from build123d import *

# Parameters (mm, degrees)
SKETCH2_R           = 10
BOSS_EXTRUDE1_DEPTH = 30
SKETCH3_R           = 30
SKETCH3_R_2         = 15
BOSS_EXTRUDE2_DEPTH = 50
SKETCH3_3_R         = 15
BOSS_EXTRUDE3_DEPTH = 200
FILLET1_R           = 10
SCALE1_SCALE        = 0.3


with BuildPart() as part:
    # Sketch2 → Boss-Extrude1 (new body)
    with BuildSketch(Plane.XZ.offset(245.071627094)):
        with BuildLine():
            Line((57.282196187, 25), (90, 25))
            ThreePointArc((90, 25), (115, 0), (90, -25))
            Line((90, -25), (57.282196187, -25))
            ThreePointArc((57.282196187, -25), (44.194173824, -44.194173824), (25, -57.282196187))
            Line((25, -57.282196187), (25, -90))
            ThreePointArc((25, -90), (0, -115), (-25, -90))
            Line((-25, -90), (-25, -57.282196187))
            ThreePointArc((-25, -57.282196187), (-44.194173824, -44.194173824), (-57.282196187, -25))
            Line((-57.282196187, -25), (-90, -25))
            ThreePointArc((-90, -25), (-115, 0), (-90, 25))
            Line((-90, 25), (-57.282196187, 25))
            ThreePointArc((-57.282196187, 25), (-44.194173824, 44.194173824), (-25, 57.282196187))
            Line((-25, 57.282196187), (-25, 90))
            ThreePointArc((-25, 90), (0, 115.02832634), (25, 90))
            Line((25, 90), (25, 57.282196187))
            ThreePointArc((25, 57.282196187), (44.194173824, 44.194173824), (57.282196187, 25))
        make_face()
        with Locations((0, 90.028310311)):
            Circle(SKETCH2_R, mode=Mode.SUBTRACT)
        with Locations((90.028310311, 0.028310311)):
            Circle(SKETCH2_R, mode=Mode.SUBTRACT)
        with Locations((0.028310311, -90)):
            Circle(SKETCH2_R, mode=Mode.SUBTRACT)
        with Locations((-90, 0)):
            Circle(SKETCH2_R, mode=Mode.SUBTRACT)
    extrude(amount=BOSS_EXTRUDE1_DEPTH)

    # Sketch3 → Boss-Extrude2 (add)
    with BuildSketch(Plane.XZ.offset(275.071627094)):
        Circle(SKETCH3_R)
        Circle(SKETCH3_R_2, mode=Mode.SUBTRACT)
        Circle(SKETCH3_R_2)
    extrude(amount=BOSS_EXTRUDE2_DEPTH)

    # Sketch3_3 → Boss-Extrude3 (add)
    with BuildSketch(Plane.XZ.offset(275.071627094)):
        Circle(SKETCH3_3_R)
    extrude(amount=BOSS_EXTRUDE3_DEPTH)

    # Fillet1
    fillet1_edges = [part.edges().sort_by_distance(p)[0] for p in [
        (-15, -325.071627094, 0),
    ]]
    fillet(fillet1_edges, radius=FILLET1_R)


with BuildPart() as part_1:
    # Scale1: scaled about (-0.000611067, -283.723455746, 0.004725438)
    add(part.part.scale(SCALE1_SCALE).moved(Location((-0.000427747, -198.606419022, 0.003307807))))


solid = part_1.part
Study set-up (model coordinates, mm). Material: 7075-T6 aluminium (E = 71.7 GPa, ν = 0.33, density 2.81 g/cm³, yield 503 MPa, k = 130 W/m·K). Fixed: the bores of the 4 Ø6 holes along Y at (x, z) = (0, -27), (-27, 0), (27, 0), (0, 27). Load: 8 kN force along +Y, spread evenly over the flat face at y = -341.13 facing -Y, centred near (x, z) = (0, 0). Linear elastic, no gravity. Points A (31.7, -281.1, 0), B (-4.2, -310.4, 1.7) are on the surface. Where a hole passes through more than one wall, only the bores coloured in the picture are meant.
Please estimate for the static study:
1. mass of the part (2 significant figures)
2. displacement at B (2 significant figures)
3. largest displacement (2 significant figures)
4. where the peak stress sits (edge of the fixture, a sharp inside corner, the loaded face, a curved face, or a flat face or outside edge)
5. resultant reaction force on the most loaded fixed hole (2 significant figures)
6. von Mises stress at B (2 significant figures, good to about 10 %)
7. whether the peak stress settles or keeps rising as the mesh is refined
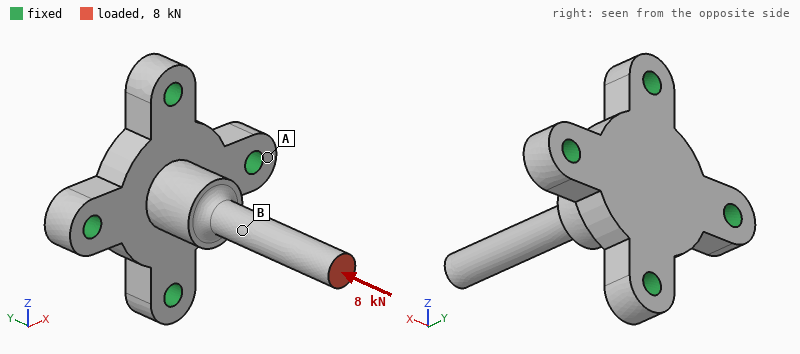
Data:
66 g
0.060 mm
0.11 mm
edge of the fixture
2.0 kN
130 MPa
keeps rising
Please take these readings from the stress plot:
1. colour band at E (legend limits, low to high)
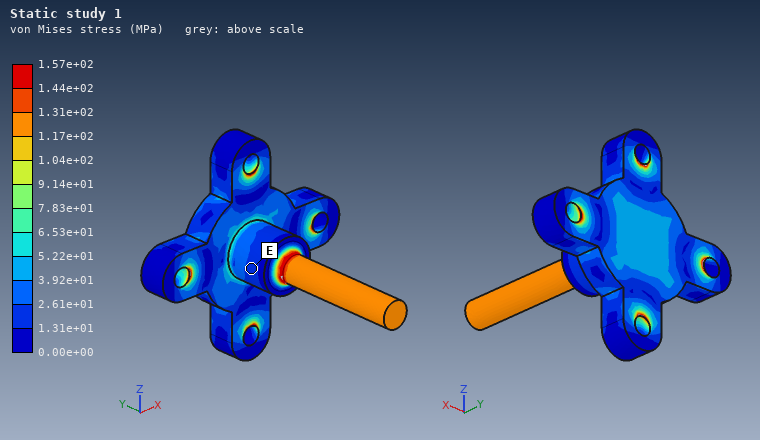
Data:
1.31e+01 to 2.61e+01 MPa
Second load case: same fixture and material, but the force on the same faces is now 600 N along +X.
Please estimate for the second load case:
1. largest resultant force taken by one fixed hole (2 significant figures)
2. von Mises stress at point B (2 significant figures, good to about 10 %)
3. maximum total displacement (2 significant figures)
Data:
910 N
240 MPa
0.93 mm
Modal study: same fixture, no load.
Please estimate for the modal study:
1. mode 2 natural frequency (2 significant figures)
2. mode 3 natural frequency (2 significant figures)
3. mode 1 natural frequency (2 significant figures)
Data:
2800 Hz
12 kHz
2800 Hz
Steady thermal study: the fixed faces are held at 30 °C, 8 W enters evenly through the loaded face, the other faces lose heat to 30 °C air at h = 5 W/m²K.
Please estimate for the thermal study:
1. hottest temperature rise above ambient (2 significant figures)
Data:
49 K
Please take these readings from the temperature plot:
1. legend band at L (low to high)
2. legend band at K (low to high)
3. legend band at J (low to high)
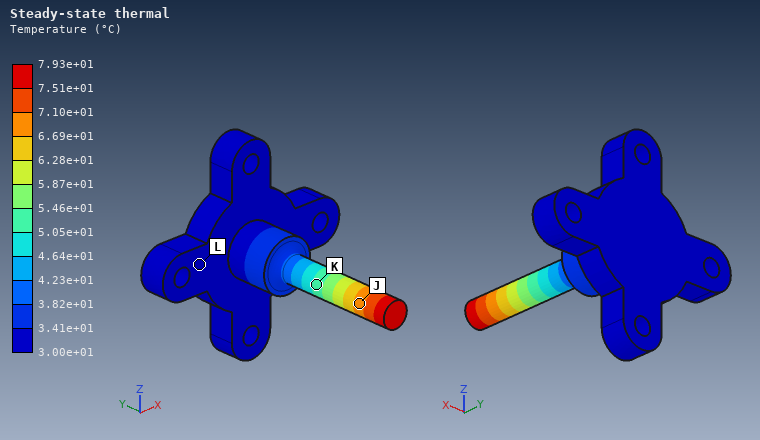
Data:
3.00e+01 to 3.41e+01 °C
5.05e+01 to 5.46e+01 °C
6.69e+01 to 7.10e+01 °C
